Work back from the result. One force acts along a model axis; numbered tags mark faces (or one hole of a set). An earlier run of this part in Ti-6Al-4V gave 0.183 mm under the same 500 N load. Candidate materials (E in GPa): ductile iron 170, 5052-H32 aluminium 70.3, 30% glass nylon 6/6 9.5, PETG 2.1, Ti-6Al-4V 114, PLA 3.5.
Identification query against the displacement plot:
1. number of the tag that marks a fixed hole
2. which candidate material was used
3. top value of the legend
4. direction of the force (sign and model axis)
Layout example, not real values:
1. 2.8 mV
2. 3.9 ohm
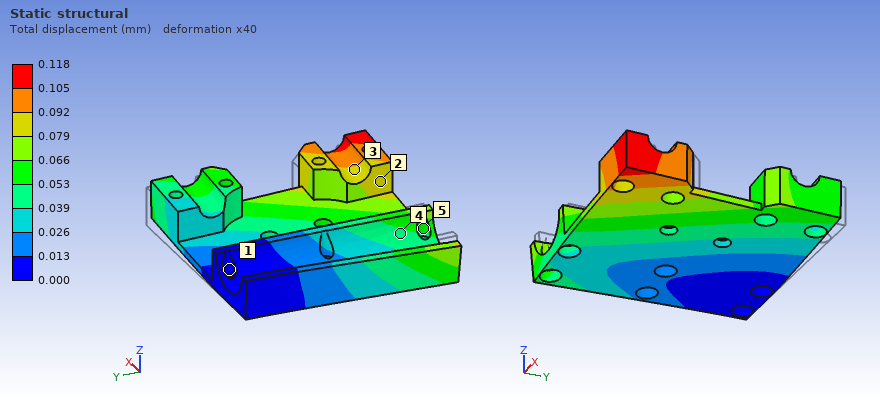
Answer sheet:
1. 1
2. ductile iron
3. 0.118 mm
4. -X
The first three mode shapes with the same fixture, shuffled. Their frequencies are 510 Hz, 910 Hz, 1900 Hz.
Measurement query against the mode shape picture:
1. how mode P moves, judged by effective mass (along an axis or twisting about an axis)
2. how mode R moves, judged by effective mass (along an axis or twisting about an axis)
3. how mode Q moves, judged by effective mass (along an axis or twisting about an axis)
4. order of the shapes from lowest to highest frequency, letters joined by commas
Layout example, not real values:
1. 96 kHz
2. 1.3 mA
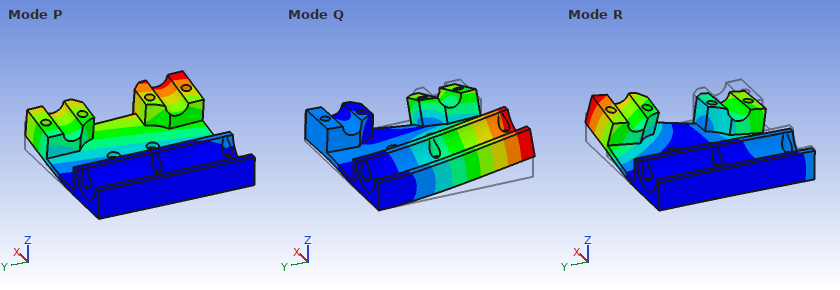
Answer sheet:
1. along Z
2. twisting about X
3. along Z
4. P, R, Q
